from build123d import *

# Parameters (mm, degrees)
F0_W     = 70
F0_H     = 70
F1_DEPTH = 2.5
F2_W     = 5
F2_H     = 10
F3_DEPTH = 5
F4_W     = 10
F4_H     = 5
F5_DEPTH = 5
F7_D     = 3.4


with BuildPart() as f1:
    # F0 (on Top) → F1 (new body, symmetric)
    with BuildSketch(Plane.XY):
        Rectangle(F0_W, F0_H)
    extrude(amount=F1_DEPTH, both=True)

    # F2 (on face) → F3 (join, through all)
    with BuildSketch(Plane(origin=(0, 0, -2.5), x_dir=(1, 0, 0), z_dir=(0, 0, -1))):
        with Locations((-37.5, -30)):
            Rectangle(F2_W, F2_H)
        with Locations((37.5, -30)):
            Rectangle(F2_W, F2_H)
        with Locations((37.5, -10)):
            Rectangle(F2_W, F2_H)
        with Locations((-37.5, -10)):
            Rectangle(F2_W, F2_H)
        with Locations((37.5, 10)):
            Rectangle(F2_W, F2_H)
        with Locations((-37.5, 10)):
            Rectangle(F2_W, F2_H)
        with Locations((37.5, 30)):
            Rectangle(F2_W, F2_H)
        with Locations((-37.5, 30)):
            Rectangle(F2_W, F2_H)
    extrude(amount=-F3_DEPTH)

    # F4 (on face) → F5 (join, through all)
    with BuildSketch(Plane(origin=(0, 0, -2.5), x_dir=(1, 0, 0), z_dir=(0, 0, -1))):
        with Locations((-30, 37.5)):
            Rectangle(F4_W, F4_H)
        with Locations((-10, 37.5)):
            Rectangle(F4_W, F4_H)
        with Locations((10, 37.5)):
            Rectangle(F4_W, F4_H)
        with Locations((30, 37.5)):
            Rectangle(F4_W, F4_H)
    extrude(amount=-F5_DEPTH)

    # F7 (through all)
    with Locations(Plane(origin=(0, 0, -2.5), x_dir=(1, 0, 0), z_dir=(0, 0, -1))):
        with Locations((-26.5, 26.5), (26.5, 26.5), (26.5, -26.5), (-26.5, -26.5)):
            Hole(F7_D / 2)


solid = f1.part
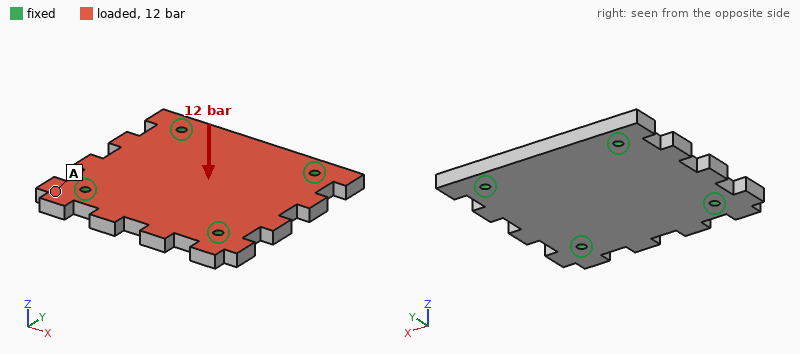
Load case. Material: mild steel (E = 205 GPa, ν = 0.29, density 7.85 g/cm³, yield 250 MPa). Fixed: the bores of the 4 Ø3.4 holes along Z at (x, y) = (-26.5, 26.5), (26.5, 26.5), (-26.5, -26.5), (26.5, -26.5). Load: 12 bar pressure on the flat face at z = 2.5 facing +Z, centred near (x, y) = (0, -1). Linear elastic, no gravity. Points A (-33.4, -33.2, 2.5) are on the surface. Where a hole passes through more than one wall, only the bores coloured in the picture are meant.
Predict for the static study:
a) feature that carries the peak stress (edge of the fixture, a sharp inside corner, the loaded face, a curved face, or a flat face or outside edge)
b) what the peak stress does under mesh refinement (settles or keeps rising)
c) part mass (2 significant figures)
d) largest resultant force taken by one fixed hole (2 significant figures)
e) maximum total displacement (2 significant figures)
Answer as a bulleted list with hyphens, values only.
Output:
- edge of the fixture
- keeps rising
- 210 g
- 1.7 kN
- 32 µm
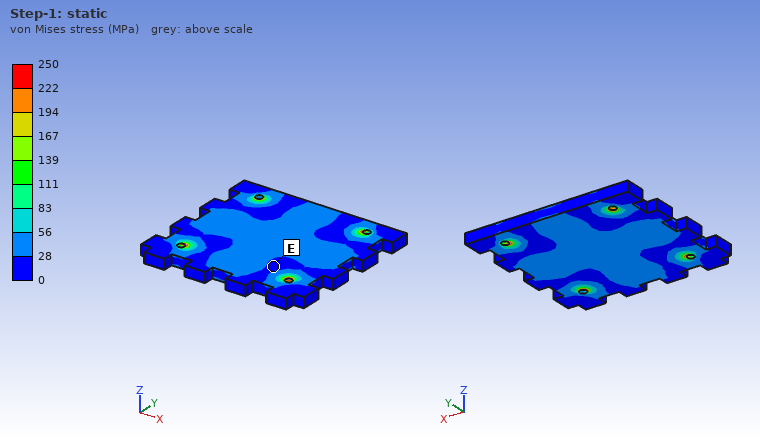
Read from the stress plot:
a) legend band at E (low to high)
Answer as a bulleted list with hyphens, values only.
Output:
- 0 to 28 MPa
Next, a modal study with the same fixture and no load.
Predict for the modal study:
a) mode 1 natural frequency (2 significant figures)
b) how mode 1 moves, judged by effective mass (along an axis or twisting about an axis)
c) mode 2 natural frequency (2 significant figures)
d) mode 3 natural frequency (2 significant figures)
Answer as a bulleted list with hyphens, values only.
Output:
- 5900 Hz
- along Z
- 8100 Hz
- 8300 Hz
